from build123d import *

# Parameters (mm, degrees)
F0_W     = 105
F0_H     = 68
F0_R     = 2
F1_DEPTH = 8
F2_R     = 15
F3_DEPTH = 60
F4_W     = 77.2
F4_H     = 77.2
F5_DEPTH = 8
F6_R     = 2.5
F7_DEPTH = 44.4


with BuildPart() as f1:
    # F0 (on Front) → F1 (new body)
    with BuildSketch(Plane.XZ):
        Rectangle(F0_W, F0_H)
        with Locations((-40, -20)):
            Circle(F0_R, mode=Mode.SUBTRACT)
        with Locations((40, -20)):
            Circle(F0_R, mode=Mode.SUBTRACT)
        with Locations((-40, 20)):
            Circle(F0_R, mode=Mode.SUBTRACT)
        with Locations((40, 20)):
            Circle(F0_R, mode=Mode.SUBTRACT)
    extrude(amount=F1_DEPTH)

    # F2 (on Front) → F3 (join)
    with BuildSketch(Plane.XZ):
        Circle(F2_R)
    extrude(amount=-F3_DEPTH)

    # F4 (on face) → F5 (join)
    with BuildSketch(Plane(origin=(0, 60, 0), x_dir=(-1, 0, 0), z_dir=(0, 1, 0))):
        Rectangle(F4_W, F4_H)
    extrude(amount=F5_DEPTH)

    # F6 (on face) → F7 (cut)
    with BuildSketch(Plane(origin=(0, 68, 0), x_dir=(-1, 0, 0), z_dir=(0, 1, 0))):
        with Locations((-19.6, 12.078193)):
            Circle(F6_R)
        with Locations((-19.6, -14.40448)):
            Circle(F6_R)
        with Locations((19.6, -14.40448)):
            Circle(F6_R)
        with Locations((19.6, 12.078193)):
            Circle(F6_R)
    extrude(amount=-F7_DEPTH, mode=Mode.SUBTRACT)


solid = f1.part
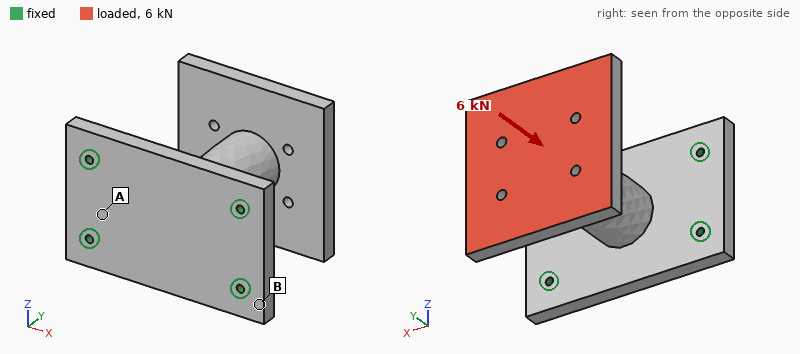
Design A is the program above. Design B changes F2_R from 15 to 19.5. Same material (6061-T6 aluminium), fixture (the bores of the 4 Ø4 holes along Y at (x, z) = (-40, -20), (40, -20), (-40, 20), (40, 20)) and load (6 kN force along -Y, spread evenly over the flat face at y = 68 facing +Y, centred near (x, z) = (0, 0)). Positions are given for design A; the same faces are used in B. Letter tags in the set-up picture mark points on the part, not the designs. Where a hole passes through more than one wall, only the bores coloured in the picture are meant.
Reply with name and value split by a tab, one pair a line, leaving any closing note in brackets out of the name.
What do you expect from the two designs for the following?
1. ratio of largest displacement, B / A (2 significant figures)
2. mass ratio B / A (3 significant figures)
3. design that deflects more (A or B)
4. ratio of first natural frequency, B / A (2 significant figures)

ratio of largest displacement, B / A	0.69
mass ratio B / A	1.20
design that deflects more	A
ratio of first natural frequency, B / A	1.1
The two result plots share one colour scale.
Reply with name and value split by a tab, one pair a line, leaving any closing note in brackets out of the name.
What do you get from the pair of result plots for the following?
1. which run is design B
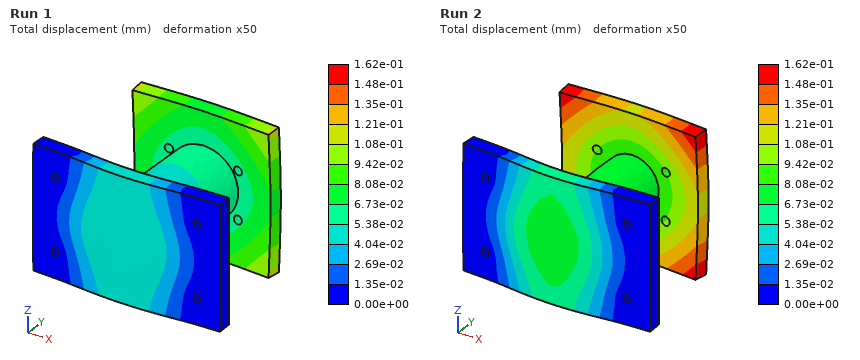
which run is design B	Run 1
